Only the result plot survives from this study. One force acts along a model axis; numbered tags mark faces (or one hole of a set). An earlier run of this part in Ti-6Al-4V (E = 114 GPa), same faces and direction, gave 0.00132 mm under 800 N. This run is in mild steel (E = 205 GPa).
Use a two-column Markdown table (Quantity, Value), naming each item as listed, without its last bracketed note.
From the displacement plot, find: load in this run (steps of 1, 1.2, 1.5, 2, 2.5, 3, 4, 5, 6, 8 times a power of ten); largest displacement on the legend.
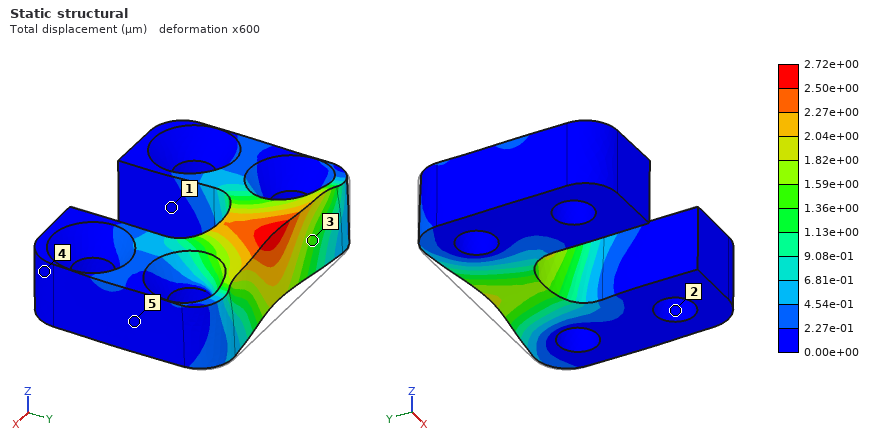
| Quantity | Value |
|---|---|
| load in this run | 3 kN |
| largest displacement on the legend | 2.72e+00 µm |
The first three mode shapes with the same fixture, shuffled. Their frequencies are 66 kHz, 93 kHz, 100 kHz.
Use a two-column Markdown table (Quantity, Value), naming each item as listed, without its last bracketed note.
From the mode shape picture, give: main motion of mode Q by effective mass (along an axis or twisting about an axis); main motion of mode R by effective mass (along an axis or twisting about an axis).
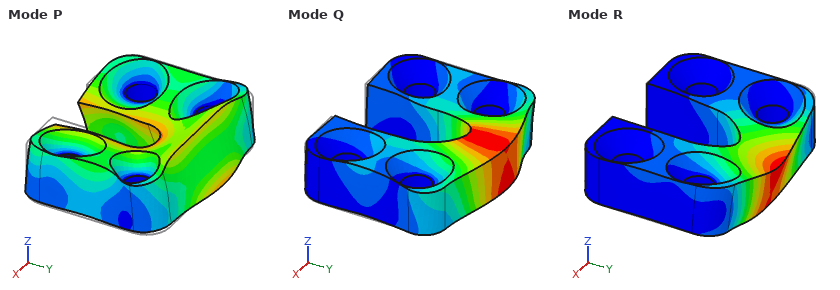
| Quantity | Value |
|---|---|
| main motion of mode Q by effective mass | along Y |
| main motion of mode R by effective mass | along Z |
